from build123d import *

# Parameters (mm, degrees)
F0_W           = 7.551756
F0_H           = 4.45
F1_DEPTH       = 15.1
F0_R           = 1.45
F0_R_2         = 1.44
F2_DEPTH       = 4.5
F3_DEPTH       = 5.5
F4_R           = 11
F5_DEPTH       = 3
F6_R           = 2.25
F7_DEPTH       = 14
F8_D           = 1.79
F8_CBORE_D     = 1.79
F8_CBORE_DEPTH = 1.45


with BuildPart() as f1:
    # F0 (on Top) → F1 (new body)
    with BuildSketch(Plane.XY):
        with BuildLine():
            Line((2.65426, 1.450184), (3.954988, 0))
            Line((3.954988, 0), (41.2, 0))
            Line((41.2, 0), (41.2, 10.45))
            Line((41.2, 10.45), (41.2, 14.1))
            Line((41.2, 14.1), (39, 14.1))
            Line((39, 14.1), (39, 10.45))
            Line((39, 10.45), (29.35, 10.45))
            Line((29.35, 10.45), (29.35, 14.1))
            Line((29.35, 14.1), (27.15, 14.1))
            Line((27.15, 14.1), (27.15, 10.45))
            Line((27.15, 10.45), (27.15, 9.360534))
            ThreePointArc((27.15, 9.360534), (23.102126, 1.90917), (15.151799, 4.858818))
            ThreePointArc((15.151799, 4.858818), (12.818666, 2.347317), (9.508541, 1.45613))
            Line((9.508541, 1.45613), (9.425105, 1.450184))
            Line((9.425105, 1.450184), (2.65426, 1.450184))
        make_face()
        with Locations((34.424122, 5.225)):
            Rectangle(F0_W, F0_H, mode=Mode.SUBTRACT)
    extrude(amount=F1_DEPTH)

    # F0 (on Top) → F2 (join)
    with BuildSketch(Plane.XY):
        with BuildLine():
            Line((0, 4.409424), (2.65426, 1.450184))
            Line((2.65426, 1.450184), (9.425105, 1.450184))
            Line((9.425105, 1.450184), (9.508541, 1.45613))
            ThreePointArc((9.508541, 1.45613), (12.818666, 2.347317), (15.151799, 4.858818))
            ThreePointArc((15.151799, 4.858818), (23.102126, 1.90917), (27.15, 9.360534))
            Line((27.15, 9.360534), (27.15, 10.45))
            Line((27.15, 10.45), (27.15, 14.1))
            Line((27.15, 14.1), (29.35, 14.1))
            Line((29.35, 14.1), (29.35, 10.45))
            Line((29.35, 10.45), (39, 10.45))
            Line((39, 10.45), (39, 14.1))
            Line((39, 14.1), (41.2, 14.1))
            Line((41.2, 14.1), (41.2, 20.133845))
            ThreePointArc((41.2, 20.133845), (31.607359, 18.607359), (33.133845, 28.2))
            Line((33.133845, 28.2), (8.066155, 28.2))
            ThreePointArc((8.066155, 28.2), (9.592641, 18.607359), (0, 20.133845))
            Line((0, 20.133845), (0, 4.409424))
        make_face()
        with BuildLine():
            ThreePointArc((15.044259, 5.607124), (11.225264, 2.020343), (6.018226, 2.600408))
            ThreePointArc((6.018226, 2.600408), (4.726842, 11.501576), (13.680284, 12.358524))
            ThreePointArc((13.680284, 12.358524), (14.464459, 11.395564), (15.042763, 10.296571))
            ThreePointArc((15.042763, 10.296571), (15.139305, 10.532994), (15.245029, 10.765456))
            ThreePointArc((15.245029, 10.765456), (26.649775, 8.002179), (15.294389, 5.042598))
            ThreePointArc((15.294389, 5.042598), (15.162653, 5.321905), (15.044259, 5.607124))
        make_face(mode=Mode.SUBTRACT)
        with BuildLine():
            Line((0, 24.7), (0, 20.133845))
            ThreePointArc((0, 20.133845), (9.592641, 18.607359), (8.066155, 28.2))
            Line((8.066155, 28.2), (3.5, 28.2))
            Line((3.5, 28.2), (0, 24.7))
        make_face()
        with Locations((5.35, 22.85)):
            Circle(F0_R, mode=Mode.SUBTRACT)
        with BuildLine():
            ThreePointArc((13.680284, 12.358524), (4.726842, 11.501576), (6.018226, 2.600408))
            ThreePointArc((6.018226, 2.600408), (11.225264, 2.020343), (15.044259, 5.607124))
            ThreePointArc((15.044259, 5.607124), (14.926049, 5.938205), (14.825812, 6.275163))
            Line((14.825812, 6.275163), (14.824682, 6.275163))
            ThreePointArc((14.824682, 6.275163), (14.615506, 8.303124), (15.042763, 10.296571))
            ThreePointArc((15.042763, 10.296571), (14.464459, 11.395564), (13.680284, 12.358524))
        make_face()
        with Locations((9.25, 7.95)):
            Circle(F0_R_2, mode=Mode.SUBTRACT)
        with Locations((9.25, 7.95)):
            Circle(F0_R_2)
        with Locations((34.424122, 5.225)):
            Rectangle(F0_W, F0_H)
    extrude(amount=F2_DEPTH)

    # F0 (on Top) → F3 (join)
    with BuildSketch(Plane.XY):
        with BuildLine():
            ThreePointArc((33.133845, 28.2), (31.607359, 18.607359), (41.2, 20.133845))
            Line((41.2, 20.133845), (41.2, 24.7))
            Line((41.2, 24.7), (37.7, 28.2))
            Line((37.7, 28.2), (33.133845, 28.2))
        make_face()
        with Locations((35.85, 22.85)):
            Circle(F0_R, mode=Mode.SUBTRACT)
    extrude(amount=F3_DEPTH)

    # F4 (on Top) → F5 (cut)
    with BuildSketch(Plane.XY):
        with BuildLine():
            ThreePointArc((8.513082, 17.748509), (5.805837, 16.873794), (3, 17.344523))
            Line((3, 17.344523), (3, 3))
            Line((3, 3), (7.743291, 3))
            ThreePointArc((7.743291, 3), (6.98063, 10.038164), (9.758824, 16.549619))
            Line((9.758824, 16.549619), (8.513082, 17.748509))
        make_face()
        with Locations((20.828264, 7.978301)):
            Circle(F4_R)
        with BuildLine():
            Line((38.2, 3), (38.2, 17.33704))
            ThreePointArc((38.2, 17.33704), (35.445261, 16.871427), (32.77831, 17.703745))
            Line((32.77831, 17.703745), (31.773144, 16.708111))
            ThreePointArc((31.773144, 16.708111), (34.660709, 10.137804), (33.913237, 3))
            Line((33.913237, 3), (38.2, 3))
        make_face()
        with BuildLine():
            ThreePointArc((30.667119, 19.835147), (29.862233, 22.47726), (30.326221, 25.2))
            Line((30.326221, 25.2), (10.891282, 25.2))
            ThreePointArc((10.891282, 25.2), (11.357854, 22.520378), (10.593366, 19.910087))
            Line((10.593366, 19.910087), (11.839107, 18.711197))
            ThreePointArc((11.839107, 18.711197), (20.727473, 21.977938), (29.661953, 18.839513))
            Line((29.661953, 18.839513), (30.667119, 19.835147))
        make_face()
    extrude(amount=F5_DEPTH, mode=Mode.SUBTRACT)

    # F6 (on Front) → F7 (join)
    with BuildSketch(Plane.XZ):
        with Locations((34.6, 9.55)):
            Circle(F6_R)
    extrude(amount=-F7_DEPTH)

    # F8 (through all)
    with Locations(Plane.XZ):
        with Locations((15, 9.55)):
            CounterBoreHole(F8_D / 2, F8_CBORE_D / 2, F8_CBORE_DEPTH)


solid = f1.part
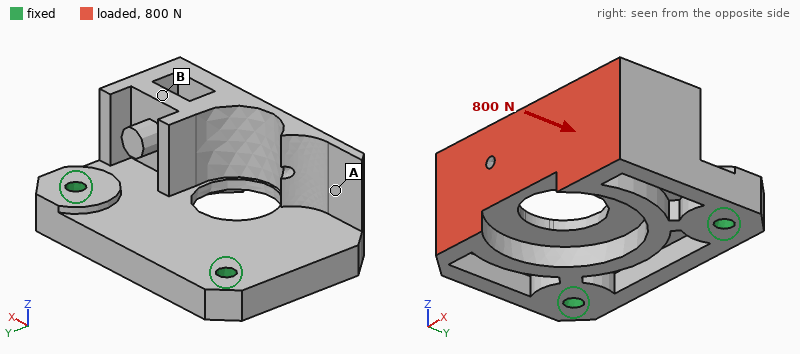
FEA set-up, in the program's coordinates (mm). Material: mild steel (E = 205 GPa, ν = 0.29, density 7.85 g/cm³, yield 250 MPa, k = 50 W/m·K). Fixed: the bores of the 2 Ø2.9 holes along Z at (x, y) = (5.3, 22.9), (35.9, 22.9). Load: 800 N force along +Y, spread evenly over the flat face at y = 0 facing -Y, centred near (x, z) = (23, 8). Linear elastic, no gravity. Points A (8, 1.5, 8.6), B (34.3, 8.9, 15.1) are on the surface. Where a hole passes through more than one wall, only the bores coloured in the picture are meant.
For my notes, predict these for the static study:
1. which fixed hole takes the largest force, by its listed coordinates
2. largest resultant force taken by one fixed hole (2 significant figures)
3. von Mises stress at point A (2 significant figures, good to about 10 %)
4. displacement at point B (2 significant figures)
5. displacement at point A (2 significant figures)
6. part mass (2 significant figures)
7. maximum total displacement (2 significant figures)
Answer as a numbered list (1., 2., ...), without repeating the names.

1. (35.9, 22.9)
2. 470 N
3. 34 MPa
4. 29 µm
5. 32 µm
6. 42 g
7. 63 µm
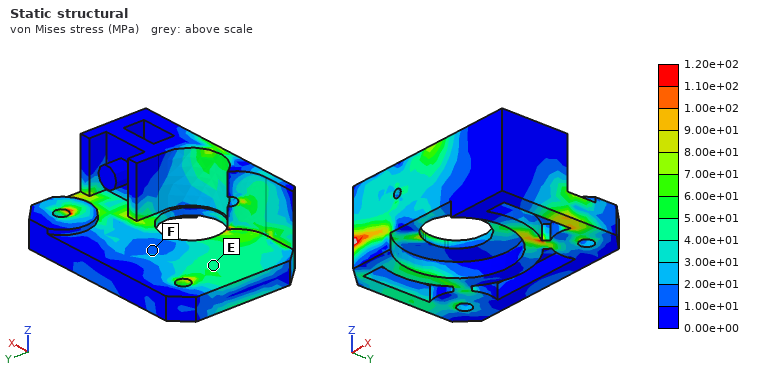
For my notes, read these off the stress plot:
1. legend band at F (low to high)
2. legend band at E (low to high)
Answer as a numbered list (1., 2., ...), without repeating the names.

1. 1.00e+01 to 2.00e+01 MPa
2. 4.00e+01 to 5.00e+01 MPa
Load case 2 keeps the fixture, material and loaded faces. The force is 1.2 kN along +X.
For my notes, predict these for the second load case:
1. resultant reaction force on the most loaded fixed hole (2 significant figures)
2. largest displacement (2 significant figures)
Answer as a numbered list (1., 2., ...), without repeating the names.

1. 1.0 kN
2. 24 µm
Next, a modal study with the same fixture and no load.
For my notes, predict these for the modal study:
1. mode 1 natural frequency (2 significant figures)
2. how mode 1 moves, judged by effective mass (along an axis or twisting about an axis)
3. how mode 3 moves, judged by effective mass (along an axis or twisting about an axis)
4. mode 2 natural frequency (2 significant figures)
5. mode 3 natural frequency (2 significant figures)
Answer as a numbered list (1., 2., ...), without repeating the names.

1. 3500 Hz
2. along Z
3. along X
4. 6600 Hz
5. 12 kHz
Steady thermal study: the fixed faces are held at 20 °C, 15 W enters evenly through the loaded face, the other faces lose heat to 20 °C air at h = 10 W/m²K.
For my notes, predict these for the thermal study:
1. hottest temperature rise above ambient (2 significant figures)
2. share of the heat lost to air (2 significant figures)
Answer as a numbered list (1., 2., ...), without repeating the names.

1. 76 K
2. 9.4 %
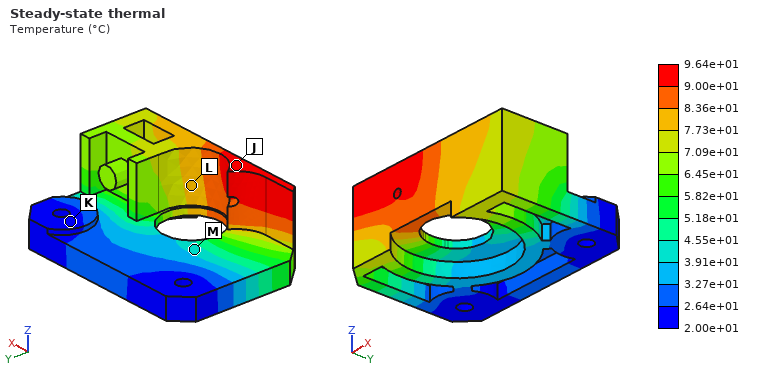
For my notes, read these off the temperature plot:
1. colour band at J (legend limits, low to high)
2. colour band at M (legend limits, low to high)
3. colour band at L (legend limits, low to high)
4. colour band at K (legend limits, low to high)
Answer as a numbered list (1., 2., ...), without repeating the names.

1. 9.00e+01 to 9.64e+01 °C
2. 3.91e+01 to 4.55e+01 °C
3. 7.73e+01 to 8.36e+01 °C
4. 2.00e+01 to 2.64e+01 °C
